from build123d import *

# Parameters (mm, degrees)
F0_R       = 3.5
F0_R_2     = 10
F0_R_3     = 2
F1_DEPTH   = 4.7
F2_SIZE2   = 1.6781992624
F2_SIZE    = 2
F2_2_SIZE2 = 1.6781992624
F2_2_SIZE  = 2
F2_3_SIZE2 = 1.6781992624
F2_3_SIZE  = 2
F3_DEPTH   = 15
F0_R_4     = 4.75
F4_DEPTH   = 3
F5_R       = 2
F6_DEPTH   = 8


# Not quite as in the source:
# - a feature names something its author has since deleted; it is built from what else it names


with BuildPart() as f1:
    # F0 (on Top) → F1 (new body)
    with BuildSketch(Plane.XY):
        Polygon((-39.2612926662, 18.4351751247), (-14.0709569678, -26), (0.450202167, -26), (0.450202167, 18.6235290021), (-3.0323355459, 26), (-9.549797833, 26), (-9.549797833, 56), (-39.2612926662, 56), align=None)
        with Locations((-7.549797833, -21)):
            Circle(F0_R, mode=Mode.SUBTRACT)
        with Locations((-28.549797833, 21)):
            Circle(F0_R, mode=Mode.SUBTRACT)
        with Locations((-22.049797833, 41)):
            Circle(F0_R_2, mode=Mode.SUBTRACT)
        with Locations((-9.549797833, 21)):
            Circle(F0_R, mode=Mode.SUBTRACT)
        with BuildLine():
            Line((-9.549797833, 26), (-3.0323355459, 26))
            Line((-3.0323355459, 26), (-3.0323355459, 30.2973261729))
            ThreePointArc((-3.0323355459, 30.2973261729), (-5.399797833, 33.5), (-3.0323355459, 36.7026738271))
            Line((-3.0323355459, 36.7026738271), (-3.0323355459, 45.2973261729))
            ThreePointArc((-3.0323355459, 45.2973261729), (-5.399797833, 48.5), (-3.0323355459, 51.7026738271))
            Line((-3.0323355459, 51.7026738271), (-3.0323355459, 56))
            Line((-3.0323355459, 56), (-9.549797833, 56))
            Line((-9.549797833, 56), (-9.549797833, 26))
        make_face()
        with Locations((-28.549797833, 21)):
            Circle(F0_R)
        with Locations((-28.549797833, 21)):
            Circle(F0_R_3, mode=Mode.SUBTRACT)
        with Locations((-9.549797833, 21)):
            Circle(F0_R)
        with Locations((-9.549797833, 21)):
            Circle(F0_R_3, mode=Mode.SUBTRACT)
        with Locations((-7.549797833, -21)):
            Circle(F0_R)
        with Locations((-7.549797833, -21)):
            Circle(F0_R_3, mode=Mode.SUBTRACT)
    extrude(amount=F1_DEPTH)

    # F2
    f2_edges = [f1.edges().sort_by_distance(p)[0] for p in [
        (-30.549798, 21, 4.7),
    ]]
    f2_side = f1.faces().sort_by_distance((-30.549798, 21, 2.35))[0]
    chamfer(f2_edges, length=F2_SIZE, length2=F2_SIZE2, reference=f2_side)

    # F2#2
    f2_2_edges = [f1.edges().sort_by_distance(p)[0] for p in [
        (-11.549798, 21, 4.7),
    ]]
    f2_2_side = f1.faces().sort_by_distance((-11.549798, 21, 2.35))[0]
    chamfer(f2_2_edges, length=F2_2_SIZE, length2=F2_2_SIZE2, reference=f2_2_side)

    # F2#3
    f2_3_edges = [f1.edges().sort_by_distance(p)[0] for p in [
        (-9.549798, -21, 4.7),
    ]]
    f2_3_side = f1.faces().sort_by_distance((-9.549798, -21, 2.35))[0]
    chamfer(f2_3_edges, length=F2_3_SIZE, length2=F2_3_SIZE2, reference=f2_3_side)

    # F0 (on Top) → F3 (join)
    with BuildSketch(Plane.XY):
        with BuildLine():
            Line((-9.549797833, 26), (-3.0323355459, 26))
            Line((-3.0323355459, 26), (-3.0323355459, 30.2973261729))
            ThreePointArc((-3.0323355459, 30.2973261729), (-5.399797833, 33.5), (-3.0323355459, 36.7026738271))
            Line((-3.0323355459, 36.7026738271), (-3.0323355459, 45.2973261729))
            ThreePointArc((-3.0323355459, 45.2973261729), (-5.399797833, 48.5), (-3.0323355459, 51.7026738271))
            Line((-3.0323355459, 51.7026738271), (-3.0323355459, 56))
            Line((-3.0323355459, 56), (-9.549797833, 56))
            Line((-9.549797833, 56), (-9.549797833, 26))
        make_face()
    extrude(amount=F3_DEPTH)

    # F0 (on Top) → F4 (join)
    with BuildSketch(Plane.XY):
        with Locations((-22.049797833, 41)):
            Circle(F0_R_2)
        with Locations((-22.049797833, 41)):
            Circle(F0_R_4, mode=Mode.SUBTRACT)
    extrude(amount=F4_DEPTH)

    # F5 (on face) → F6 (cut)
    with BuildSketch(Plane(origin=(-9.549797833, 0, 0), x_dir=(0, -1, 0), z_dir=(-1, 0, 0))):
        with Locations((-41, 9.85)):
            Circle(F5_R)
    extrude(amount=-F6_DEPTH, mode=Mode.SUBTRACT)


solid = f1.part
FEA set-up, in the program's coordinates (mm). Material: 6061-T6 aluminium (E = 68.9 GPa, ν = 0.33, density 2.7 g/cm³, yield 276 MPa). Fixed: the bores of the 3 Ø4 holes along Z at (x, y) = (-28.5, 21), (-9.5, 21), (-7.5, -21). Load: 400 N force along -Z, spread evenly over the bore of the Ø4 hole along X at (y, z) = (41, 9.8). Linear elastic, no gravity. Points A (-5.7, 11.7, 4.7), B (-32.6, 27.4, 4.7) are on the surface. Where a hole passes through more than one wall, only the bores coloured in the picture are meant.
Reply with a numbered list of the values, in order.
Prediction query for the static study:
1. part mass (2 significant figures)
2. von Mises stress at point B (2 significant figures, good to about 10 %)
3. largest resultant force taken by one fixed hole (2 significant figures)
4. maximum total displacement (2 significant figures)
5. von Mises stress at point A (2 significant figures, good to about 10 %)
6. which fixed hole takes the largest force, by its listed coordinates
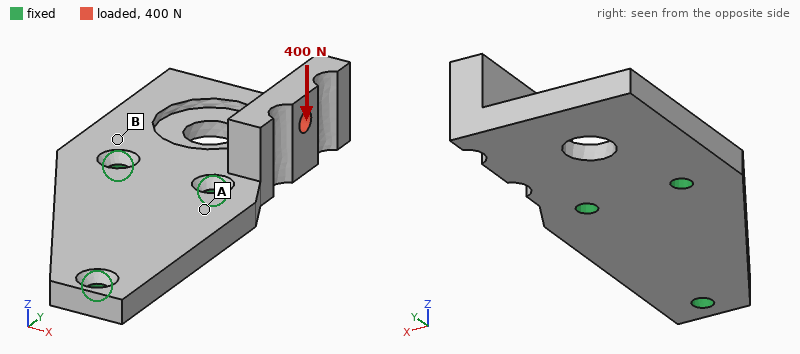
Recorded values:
1. 34 g
2. 28 MPa
3. 490 N
4. 0.20 mm
5. 13 MPa
6. (-9.5, 21)
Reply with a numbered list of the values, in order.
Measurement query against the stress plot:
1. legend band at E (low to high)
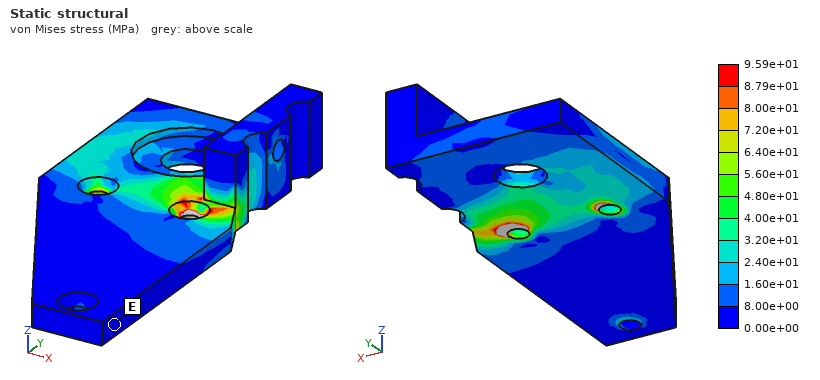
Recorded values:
1. 0.00e+00 to 8.00e+00 MPa
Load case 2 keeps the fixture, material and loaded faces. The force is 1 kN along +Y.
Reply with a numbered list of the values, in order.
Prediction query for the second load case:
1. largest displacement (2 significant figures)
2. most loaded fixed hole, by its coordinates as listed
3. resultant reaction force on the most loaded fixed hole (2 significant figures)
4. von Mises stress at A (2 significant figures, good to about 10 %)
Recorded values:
1. 0.23 mm
2. (-9.5, 21)
3. 840 N
4. 15 MPa
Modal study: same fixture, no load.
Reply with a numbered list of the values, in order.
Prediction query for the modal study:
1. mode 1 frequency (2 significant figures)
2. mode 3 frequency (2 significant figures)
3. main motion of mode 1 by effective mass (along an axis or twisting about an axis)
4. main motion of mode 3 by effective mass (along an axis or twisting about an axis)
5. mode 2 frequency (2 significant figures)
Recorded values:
1. 2500 Hz
2. 9500 Hz
3. along Z
4. along X
5. 4900 Hz
